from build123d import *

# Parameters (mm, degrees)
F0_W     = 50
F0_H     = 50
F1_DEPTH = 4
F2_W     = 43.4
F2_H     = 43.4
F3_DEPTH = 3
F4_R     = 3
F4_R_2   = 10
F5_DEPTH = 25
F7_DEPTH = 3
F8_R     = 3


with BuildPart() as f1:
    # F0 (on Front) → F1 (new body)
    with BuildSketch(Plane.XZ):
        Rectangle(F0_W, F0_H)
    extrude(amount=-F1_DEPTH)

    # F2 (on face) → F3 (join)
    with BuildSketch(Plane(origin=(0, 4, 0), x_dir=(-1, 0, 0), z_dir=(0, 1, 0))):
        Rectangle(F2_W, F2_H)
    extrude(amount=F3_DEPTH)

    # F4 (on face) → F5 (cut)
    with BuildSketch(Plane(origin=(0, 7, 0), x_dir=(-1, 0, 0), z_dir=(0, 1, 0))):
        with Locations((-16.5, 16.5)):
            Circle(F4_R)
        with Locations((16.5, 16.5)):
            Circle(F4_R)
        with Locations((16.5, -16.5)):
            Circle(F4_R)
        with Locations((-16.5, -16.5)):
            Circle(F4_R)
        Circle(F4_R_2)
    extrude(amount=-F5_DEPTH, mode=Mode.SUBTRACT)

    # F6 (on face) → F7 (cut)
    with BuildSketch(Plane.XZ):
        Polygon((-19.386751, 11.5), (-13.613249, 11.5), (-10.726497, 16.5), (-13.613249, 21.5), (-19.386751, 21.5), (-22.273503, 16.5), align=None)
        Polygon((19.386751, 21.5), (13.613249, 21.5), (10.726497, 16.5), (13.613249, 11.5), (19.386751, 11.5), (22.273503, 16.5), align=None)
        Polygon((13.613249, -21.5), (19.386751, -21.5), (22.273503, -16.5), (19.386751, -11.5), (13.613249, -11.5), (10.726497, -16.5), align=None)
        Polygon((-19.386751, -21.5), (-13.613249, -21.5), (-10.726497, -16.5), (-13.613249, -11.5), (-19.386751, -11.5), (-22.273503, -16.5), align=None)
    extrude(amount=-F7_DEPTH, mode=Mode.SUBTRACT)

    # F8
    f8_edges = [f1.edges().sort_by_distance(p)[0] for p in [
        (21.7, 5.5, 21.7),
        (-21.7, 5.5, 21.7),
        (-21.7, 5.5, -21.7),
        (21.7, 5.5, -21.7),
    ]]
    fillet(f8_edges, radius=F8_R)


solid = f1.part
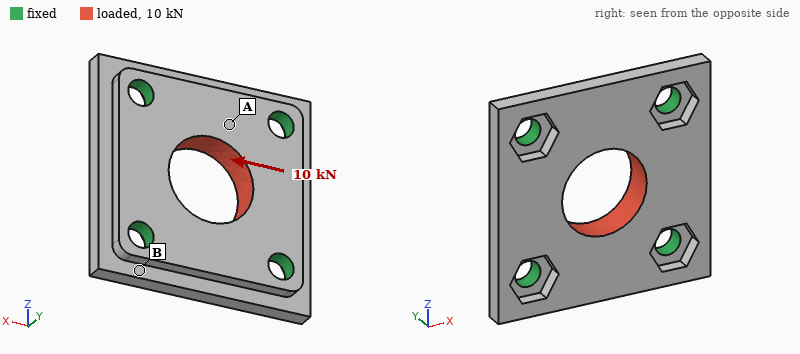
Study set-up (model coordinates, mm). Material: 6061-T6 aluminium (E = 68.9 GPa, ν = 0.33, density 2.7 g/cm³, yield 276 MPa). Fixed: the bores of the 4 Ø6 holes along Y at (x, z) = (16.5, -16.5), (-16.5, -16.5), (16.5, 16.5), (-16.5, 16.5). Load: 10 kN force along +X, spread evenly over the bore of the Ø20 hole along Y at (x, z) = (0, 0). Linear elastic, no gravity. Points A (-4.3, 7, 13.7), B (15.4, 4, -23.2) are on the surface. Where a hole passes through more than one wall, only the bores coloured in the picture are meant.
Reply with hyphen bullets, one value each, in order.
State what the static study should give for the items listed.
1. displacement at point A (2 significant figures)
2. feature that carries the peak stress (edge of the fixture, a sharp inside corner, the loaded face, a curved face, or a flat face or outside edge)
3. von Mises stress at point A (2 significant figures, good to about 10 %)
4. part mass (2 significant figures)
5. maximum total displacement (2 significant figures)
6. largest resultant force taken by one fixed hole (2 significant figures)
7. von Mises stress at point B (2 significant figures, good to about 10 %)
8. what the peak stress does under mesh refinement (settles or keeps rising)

- 5.3 µm
- edge of the fixture
- 35 MPa
- 32 g
- 13 µm
- 2.6 kN
- 13 MPa
- keeps rising
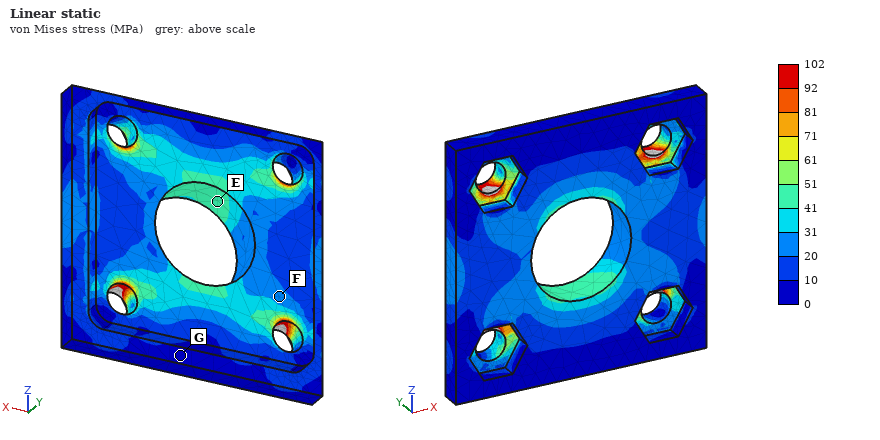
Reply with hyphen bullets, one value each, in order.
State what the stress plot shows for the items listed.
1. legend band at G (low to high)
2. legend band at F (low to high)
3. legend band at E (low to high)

- 0 to 10 MPa
- 20 to 31 MPa
- 41 to 51 MPa
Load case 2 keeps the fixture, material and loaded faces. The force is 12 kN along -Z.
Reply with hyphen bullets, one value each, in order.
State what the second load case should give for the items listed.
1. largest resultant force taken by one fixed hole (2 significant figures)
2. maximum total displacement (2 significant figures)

- 3.1 kN
- 16 µm
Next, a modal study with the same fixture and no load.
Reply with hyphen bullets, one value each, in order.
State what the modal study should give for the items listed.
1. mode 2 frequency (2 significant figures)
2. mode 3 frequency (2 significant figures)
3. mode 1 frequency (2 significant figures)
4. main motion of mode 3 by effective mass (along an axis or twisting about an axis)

- 23 kHz
- 25 kHz
- 22 kHz
- twisting about X
